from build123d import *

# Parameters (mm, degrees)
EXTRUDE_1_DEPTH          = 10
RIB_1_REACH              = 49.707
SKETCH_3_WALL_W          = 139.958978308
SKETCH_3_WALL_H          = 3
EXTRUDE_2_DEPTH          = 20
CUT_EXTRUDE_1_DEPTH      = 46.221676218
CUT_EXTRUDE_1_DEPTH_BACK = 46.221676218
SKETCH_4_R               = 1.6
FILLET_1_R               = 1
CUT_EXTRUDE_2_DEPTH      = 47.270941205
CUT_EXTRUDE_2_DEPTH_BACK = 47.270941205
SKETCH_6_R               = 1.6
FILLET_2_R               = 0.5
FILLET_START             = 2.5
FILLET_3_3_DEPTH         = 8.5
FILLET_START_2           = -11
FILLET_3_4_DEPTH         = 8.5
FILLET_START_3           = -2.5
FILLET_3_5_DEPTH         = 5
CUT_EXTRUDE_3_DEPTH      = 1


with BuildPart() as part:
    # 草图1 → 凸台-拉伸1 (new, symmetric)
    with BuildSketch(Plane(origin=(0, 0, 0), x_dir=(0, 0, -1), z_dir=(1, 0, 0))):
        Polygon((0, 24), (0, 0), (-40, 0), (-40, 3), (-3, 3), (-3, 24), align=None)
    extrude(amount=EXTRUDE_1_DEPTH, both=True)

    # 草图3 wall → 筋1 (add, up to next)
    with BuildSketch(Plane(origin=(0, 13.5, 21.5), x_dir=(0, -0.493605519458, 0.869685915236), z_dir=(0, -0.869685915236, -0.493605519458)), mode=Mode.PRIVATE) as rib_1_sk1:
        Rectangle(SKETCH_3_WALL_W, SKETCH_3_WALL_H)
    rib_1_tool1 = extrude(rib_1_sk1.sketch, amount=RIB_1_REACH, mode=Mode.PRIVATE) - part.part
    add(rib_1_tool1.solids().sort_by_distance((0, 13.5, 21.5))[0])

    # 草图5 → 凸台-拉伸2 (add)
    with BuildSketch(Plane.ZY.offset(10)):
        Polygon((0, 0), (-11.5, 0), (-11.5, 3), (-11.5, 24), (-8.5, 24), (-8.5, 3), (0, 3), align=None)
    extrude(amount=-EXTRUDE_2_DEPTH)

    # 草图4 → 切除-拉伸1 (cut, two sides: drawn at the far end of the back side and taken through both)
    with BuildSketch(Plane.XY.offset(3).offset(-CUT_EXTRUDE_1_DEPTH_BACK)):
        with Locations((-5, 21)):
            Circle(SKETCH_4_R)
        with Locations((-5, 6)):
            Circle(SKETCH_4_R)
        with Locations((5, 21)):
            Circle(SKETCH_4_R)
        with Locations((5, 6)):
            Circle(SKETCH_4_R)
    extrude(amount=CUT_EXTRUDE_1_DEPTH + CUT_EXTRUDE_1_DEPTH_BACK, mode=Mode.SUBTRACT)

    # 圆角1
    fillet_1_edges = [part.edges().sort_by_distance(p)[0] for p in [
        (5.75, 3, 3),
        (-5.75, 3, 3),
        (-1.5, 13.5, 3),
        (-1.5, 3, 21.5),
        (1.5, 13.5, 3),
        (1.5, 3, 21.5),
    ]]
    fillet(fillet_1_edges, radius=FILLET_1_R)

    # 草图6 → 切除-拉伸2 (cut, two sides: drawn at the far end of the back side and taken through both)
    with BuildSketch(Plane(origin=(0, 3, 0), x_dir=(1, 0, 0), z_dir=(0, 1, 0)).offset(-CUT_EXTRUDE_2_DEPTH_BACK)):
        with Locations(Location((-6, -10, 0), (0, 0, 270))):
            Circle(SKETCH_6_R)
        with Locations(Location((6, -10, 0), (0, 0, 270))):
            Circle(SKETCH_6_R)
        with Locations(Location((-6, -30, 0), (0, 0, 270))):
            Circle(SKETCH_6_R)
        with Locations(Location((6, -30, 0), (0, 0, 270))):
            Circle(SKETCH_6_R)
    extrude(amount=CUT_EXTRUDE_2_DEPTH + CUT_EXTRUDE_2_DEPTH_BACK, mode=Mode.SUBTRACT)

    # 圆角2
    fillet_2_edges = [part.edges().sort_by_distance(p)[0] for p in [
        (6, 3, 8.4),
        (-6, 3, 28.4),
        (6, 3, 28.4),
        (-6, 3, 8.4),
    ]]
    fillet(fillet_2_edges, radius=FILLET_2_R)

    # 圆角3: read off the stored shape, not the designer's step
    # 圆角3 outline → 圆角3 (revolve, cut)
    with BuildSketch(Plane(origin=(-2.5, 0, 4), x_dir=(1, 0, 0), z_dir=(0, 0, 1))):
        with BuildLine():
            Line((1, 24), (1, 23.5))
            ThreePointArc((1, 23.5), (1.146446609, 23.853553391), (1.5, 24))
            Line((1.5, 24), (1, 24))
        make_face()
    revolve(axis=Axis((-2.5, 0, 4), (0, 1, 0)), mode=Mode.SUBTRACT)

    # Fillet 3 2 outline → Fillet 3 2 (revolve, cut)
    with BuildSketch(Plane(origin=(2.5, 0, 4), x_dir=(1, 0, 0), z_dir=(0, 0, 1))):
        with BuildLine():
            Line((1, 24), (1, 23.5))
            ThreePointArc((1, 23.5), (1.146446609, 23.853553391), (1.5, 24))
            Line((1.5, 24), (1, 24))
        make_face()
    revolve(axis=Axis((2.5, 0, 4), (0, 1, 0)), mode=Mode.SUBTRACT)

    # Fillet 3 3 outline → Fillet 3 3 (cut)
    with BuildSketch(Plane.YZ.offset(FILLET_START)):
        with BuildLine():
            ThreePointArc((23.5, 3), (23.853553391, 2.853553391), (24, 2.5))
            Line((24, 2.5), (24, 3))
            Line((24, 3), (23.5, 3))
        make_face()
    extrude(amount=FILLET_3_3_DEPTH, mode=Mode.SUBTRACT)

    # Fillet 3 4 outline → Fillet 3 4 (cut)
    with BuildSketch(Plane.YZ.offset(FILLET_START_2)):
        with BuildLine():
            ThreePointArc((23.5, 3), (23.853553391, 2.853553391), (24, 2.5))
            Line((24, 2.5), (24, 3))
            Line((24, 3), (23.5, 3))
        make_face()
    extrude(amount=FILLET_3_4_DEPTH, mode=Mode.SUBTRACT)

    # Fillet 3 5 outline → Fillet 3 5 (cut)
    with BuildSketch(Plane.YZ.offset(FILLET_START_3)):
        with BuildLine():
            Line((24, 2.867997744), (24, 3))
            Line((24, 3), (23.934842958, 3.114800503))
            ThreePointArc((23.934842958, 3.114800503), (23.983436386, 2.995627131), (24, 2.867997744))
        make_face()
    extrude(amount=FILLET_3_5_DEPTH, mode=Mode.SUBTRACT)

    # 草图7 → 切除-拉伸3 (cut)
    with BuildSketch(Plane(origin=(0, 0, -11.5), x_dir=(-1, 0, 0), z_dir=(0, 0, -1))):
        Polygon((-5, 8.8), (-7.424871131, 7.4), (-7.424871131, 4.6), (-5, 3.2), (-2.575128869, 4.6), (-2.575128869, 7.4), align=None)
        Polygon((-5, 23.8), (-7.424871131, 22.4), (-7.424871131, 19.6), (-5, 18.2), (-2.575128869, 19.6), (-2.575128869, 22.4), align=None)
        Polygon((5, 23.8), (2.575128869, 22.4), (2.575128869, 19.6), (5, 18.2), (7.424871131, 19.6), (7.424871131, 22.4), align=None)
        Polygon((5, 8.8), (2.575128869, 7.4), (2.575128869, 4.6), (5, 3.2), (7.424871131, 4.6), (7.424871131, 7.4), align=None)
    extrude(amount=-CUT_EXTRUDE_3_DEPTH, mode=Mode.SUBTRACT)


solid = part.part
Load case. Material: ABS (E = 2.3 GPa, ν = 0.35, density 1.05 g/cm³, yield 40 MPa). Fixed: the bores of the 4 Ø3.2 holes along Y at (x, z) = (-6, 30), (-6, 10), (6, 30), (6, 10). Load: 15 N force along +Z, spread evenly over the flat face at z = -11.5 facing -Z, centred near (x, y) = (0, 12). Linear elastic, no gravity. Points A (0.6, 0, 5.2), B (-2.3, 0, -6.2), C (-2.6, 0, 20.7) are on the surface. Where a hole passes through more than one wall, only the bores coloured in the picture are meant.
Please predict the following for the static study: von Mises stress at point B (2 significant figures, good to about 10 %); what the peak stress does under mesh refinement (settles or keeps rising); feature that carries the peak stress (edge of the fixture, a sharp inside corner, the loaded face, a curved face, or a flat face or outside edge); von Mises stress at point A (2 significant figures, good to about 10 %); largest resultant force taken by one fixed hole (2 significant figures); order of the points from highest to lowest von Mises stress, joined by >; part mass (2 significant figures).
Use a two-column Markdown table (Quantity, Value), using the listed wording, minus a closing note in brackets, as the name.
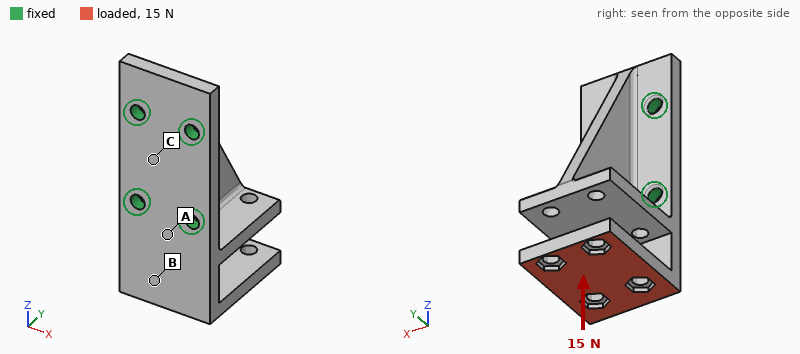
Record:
| Quantity | Value |
|---|---|
| von Mises stress at point B | 4.0 MPa |
| what the peak stress does under mesh refinement | keeps rising |
| feature that carries the peak stress | a sharp inside corner |
| von Mises stress at point A | 1.0 MPa |
| largest resultant force taken by one fixed hole | 5.8 N |
| order of the points from highest to lowest von Mises stress, joined by > | B > A > C |
| part mass | 6.8 g |
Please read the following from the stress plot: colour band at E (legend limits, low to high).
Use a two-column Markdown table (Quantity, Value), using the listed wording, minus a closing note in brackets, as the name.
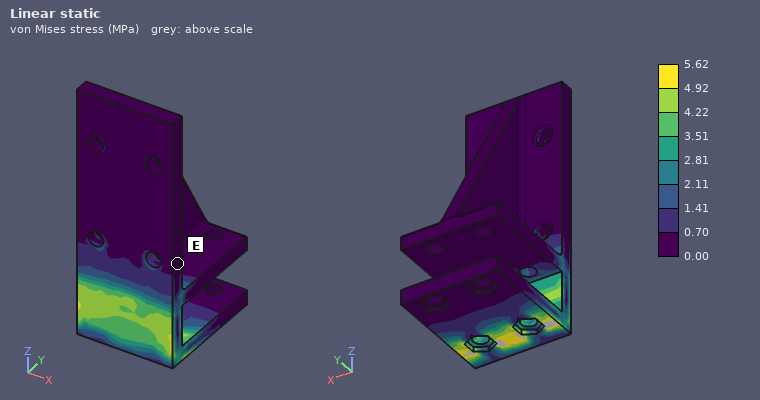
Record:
| Quantity | Value |
|---|---|
| colour band at E | 0.00 to 0.70 MPa |
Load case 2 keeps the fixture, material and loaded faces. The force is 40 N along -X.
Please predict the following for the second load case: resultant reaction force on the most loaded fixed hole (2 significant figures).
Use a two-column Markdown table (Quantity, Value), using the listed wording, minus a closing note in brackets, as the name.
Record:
| Quantity | Value |
|---|---|
| resultant reaction force on the most loaded fixed hole | 70 N |
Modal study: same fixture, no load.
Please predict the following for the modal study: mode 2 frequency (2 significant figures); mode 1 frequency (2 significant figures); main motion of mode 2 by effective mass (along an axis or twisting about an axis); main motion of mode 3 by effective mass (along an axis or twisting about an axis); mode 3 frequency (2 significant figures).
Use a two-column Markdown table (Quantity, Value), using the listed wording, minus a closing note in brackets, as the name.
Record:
| Quantity | Value |
|---|---|
| mode 2 frequency | 1200 Hz |
| mode 1 frequency | 770 Hz |
| main motion of mode 2 by effective mass | along X |
| main motion of mode 3 by effective mass | along Y |
| mode 3 frequency | 1900 Hz |
